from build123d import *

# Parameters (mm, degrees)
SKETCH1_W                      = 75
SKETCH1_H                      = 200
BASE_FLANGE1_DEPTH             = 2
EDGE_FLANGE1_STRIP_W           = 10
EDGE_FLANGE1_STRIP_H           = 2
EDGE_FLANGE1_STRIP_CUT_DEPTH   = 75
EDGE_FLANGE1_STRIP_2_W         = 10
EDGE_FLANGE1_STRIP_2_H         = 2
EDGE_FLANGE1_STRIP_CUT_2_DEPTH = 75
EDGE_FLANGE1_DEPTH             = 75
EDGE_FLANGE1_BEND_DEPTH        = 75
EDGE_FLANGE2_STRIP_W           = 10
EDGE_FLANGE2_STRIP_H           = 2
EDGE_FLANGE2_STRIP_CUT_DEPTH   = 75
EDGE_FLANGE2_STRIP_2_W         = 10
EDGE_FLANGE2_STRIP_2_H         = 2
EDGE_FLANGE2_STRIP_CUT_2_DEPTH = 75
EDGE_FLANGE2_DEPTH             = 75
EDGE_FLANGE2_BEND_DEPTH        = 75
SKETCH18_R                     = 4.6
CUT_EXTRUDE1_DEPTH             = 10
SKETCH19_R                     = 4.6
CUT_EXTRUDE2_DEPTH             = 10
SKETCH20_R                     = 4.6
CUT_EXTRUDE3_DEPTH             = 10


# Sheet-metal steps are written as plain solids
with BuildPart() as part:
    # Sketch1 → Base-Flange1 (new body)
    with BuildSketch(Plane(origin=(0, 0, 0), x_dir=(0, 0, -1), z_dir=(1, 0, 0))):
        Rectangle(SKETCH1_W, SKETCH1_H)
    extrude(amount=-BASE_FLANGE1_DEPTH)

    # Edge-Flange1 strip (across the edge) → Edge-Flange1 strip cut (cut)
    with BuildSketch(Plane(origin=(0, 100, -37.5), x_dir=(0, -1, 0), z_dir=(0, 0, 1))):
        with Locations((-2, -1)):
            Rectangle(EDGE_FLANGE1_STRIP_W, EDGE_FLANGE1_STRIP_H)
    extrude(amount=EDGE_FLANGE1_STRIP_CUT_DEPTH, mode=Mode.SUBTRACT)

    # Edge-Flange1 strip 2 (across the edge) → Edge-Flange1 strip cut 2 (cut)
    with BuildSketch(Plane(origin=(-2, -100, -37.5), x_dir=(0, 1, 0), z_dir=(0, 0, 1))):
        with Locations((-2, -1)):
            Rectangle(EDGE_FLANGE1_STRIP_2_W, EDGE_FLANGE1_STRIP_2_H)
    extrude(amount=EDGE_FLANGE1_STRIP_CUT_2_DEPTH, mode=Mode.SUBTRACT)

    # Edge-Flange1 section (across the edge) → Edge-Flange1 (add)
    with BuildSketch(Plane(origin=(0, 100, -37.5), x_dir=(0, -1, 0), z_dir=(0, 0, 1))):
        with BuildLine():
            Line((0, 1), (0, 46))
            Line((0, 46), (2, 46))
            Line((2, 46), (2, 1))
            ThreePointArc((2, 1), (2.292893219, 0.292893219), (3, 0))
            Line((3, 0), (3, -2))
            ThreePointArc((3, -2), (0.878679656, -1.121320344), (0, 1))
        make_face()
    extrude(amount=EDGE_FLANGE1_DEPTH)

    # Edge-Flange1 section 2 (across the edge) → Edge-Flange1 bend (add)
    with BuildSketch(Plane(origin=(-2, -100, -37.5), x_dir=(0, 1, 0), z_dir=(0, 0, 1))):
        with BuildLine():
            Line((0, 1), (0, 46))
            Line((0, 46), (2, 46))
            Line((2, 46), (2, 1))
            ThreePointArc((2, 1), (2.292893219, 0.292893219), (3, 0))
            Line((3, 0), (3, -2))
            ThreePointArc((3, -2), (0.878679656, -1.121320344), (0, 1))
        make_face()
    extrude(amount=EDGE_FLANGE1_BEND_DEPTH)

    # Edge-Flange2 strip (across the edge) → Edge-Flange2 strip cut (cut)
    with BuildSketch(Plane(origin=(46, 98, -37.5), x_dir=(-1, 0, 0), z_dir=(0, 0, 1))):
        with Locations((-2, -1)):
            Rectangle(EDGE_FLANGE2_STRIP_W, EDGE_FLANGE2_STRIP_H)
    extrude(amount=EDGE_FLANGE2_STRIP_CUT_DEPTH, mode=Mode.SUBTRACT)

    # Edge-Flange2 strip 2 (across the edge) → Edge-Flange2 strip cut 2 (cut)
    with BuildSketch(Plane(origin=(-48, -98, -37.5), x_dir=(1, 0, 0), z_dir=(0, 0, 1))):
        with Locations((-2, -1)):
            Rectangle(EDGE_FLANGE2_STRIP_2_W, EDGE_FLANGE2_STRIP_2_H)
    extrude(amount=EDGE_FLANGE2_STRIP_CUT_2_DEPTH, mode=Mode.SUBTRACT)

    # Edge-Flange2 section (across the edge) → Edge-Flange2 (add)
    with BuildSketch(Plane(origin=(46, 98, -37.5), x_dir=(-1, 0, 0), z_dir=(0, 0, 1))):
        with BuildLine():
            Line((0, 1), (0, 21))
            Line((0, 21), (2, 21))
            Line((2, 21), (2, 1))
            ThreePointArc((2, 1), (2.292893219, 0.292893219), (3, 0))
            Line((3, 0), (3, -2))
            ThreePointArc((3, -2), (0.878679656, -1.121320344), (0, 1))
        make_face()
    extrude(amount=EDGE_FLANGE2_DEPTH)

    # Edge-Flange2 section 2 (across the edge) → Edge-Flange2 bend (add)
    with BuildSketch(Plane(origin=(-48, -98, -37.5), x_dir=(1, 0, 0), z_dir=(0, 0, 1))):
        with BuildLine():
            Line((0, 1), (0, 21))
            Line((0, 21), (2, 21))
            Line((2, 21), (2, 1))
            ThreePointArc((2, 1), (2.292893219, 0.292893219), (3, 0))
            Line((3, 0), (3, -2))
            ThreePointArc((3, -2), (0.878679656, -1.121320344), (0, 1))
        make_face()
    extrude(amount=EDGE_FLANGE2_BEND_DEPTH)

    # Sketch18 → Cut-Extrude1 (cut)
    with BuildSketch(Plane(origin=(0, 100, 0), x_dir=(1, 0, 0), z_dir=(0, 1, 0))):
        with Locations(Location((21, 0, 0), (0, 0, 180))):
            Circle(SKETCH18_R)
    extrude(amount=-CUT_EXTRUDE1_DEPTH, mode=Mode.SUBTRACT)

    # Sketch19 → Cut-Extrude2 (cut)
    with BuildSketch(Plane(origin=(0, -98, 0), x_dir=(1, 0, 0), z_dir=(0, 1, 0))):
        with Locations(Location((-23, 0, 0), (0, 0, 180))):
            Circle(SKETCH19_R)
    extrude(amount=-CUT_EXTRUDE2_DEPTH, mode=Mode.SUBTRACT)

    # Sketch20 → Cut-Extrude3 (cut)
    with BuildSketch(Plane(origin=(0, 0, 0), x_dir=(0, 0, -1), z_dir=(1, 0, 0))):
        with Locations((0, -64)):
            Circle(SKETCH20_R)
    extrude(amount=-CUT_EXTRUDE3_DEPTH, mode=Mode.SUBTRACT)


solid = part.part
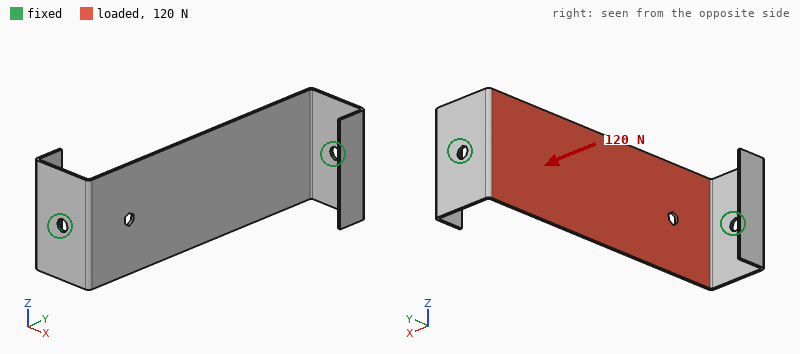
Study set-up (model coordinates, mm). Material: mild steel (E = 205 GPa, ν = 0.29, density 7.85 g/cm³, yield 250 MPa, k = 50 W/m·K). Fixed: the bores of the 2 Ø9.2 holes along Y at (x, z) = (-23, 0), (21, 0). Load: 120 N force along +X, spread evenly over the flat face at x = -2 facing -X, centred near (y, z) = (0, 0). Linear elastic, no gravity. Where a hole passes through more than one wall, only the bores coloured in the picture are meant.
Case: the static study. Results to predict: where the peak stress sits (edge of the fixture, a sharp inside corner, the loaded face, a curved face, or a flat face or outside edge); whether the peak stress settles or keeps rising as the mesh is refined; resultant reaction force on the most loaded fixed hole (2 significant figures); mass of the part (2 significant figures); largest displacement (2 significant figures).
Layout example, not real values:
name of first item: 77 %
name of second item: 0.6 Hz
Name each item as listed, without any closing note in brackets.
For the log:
where the peak stress sits: edge of the fixture
whether the peak stress settles or keeps rising as the mesh is refined: keeps rising
resultant reaction force on the most loaded fixed hole: 60 N
mass of the part: 390 g
largest displacement: 0.41 mm
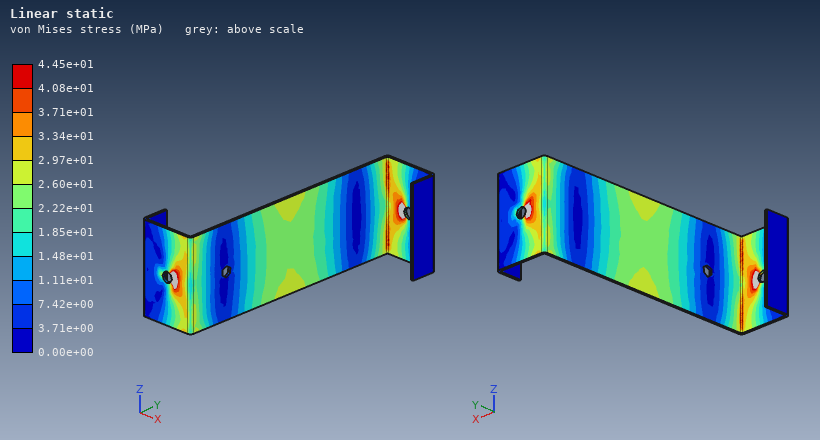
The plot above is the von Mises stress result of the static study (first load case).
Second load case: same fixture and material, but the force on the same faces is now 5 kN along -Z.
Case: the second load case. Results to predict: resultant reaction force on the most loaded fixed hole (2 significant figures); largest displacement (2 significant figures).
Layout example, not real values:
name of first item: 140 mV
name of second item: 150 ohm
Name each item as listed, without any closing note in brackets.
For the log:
resultant reaction force on the most loaded fixed hole: 2.5 kN
largest displacement: 0.25 mm
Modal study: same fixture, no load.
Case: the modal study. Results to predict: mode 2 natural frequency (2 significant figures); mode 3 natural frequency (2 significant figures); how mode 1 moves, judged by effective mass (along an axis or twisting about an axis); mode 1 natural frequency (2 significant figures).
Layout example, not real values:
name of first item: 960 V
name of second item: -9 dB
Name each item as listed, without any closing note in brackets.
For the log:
mode 2 natural frequency: 490 Hz
mode 3 natural frequency: 680 Hz
how mode 1 moves, judged by effective mass: along X
mode 1 natural frequency: 210 Hz
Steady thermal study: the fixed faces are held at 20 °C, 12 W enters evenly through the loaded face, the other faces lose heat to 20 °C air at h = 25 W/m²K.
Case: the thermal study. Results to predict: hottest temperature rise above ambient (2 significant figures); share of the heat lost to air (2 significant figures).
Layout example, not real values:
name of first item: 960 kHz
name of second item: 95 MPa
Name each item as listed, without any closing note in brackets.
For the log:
hottest temperature rise above ambient: 23 K
share of the heat lost to air: 72 %
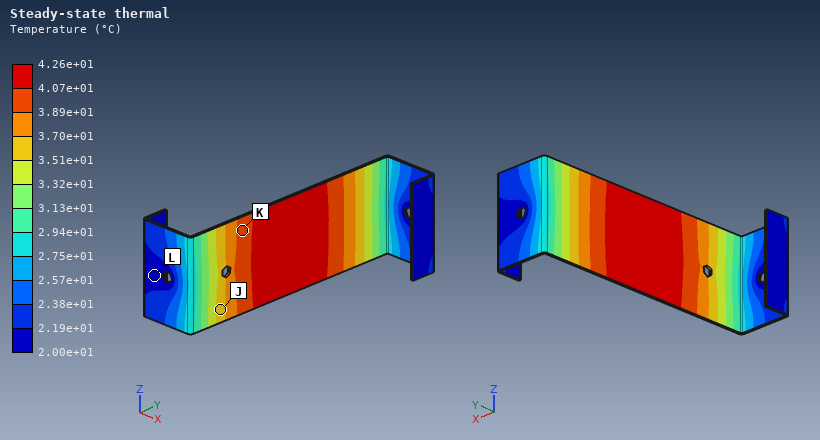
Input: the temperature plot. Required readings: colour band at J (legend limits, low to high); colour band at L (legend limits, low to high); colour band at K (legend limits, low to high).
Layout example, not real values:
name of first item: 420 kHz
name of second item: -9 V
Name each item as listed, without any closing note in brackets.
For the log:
colour band at J: 3.51e+01 to 3.70e+01 °C
colour band at L: 2.00e+01 to 2.19e+01 °C
colour band at K: 3.89e+01 to 4.07e+01 °C
